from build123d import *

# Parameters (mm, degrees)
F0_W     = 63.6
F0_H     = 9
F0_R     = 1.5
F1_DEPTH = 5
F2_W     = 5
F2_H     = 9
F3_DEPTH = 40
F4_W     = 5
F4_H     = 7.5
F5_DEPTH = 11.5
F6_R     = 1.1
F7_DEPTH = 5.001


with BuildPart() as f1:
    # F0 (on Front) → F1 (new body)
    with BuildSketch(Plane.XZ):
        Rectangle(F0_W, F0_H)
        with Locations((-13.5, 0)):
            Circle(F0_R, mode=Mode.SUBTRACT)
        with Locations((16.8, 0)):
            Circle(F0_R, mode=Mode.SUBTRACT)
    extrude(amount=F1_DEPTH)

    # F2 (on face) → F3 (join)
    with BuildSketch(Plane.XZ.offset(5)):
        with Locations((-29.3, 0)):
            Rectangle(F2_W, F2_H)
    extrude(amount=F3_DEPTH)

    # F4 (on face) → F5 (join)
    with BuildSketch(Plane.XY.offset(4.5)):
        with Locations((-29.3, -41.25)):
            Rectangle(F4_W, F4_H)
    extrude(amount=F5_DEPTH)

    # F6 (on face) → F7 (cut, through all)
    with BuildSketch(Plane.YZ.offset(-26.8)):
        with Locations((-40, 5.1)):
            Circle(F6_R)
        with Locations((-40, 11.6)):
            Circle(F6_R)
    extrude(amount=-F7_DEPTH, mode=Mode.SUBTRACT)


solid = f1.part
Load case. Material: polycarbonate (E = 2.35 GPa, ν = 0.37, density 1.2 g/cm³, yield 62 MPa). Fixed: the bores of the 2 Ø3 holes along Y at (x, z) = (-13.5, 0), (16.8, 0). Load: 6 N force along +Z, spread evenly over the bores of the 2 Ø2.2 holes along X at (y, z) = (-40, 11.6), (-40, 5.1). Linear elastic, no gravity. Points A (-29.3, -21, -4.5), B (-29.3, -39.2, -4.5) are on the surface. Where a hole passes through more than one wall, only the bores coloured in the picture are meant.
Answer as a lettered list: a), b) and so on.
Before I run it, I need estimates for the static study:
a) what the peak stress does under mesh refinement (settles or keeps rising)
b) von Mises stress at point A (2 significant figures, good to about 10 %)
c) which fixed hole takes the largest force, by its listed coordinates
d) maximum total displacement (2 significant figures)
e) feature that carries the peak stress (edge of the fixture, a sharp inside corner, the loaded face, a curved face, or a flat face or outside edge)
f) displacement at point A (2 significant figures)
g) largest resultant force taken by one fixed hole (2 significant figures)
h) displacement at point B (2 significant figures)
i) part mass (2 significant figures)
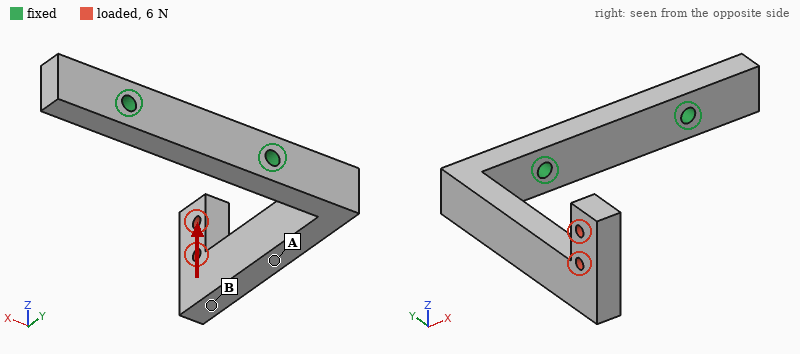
a) keeps rising
b) 1.7 MPa
c) (-13.5, 0)
d) 0.85 mm
e) edge of the fixture
f) 0.33 mm
g) 7.2 N
h) 0.68 mm
i) 6.0 g
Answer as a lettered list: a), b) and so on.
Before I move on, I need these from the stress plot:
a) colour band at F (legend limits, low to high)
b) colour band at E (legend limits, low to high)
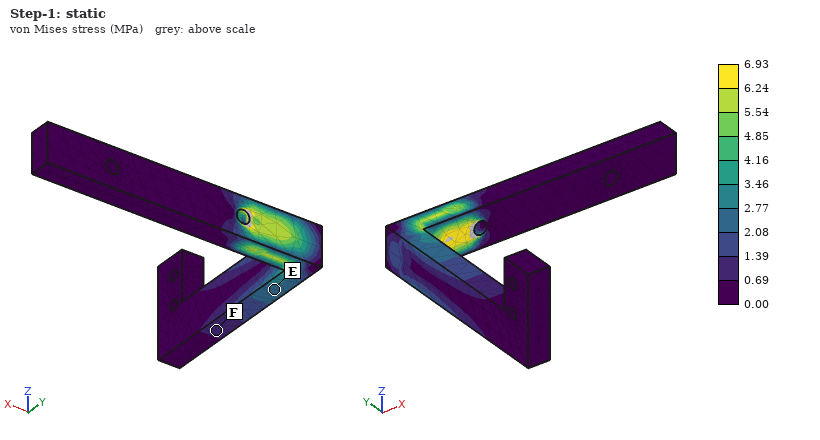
a) 0.69 to 1.39 MPa
b) 2.08 to 2.77 MPa
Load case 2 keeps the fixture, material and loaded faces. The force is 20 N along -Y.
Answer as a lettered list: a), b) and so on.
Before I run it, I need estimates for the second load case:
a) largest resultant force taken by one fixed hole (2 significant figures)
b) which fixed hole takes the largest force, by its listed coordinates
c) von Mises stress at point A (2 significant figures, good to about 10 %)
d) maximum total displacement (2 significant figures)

a) 21 N
b) (-13.5, 0)
c) 2.0 MPa
d) 0.94 mm
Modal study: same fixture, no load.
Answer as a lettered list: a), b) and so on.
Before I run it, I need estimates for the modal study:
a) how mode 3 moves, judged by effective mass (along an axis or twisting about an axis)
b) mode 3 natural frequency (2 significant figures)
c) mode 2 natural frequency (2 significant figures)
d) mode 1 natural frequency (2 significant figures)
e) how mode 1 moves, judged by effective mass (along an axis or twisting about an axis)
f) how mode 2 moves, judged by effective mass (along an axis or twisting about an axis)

a) along Y
b) 1400 Hz
c) 380 Hz
d) 320 Hz
e) along X
f) along Z
